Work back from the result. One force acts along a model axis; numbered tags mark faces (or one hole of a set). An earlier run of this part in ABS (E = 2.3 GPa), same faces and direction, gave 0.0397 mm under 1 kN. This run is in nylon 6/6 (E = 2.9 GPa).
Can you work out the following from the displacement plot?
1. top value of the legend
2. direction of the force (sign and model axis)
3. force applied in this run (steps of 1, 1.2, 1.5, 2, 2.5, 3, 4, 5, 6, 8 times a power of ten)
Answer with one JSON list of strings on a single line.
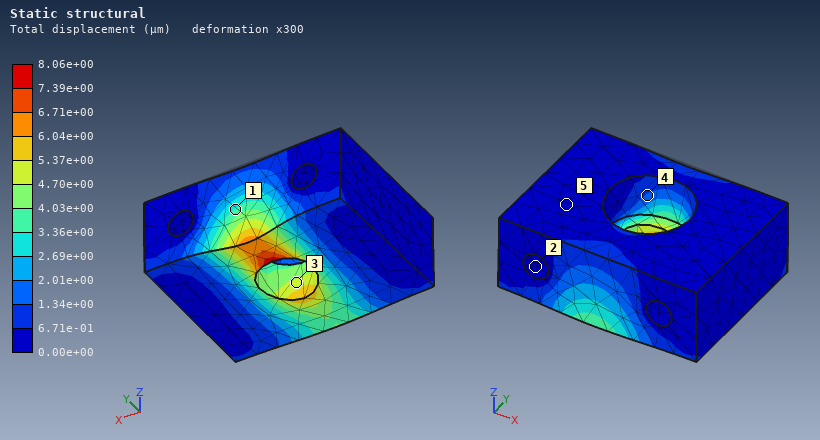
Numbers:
["8.06e+00 µm", "-Y", "250 N"]
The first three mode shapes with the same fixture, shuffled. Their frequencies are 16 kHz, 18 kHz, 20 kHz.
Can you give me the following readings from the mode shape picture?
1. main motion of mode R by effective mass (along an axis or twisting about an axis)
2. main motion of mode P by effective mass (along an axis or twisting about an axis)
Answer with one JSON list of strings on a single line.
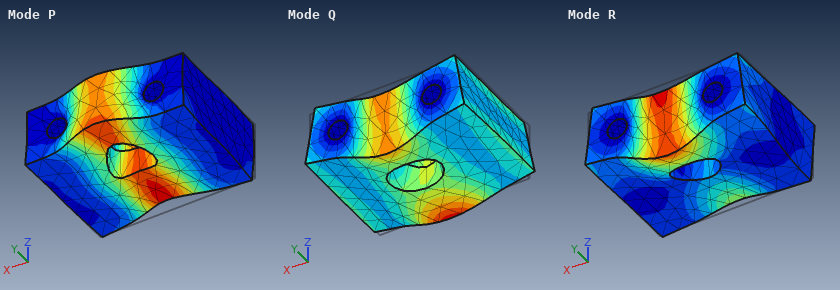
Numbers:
["twisting about X", "along Y"]
